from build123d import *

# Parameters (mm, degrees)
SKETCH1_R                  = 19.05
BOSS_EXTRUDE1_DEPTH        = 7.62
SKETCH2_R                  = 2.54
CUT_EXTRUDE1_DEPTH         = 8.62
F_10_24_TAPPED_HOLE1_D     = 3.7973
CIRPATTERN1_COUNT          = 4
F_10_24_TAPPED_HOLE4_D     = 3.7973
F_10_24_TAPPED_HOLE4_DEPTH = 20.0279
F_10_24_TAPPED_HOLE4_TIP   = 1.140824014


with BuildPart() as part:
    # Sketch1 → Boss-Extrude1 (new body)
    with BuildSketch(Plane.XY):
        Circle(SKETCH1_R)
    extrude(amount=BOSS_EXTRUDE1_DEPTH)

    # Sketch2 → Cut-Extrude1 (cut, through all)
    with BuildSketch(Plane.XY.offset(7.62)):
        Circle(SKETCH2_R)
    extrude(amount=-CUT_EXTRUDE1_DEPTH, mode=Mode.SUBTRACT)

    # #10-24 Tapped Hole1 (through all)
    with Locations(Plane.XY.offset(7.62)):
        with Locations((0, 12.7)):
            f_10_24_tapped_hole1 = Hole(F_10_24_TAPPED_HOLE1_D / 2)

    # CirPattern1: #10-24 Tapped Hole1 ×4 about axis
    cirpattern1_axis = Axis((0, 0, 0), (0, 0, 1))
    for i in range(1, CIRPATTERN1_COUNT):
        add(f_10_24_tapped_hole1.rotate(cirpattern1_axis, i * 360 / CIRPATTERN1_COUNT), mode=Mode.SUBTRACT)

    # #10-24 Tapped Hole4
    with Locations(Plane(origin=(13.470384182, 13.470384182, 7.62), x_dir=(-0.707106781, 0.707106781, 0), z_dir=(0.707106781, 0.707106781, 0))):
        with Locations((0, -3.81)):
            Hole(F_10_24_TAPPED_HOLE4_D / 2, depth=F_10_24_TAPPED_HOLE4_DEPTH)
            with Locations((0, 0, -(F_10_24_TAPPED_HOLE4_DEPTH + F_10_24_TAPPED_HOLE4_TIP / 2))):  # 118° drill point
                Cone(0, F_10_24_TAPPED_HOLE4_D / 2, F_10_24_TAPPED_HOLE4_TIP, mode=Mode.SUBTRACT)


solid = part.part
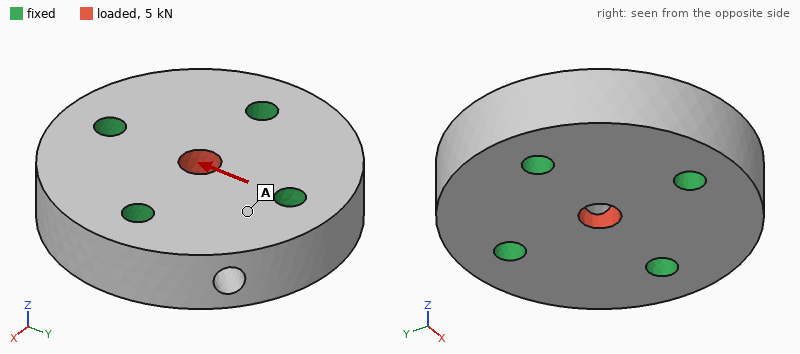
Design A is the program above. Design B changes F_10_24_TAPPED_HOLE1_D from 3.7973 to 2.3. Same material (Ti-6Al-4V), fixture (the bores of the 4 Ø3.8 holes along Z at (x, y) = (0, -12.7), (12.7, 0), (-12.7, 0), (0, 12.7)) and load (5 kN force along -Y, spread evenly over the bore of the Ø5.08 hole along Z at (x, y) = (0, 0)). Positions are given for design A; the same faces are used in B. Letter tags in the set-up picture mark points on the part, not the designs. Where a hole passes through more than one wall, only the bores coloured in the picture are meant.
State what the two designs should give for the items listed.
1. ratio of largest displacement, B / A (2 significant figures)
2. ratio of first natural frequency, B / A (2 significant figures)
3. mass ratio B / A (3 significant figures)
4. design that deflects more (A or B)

1.1
0.84
1.03
B
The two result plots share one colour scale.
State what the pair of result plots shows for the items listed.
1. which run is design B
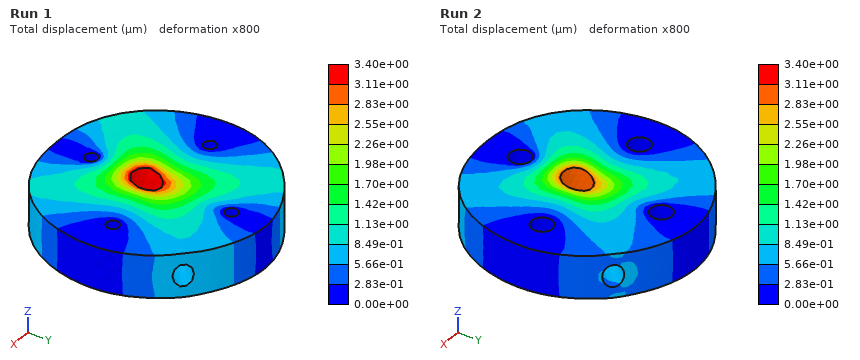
Run 1
